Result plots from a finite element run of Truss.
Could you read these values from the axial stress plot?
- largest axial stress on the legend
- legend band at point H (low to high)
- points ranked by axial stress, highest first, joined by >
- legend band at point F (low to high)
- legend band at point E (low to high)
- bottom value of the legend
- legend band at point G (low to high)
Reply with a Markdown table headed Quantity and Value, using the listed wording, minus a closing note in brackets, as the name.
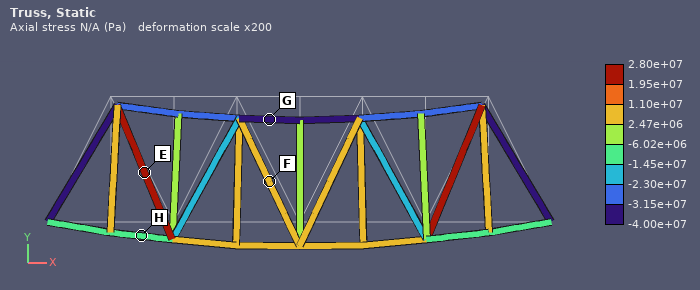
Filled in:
| Quantity | Value |
|---|---|
| largest axial stress on the legend | 2.80e+07 Pa |
| legend band at point H | -1.45e+07 to -6.02e+06 Pa |
| points ranked by axial stress, highest first, joined by > | E > F > H > G |
| legend band at point F | 2.47e+06 to 1.10e+07 Pa |
| legend band at point E | 1.95e+07 to 2.80e+07 Pa |
| bottom value of the legend | -4.00e+07 Pa |
| legend band at point G | -4.00e+07 to -3.15e+07 Pa |
